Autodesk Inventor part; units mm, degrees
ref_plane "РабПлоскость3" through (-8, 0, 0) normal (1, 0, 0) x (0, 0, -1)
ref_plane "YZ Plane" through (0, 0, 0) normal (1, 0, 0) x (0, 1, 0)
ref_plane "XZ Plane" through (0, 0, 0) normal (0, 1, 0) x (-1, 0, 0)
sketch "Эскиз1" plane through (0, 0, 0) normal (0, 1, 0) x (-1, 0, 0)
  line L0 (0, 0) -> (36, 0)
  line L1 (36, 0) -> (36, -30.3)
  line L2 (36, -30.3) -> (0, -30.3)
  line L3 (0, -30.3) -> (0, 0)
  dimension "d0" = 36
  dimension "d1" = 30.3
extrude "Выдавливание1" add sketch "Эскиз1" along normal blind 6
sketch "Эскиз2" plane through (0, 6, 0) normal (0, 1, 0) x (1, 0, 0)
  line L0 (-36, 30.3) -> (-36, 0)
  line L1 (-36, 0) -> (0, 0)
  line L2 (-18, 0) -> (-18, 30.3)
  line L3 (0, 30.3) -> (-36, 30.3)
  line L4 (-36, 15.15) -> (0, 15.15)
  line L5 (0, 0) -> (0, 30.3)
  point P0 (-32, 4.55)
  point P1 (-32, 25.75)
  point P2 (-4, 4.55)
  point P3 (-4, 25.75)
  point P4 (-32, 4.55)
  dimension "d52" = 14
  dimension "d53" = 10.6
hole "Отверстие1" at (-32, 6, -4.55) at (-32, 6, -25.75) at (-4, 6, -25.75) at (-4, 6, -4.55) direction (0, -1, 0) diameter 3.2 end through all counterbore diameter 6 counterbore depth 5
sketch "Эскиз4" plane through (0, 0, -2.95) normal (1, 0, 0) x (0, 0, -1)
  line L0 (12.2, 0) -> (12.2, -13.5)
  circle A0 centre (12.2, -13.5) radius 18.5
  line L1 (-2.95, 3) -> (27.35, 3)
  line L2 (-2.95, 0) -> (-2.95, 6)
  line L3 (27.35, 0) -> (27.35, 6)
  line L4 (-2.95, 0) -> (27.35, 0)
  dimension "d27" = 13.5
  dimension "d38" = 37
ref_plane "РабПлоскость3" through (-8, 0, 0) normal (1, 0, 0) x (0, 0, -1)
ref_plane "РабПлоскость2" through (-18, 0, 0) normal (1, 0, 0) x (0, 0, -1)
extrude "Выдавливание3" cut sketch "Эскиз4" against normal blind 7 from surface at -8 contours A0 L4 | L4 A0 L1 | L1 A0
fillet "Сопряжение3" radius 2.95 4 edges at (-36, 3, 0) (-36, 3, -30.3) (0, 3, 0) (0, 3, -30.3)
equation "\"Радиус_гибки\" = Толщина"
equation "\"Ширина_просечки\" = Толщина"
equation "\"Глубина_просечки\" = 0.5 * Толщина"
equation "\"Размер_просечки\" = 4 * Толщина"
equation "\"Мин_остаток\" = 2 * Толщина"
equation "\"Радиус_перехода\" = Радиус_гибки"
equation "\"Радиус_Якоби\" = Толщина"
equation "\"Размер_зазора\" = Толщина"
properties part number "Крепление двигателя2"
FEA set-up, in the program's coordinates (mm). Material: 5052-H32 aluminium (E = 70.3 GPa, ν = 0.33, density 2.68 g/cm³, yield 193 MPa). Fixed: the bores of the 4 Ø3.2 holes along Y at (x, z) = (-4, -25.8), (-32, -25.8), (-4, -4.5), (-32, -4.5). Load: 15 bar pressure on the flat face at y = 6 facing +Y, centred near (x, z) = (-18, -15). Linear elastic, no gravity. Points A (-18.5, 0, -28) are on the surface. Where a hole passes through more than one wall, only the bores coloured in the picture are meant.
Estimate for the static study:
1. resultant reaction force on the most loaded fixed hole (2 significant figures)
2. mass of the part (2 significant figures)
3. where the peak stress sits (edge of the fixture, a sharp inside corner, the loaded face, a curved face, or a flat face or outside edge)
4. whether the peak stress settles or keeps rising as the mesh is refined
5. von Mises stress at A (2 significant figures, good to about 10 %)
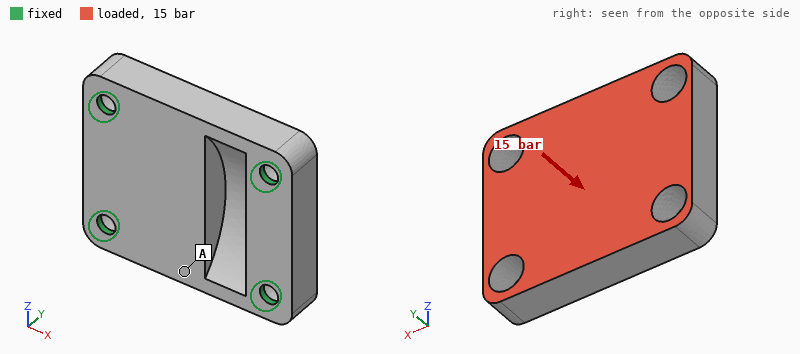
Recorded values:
460 N
14 g
edge of the fixture
keeps rising
16 MPa
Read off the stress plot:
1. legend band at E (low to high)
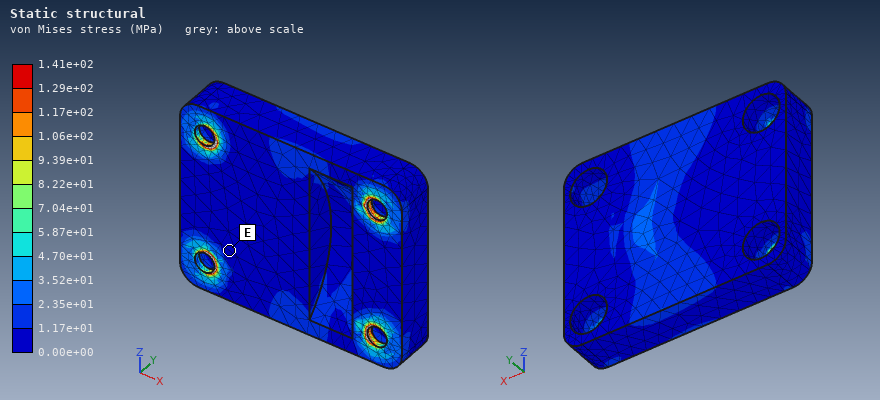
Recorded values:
0.00e+00 to 1.17e+01 MPa
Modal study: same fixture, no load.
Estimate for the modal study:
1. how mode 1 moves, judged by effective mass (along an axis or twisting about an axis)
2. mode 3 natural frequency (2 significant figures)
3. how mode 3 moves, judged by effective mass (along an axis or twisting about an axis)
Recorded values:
along Y
27 kHz
along X
